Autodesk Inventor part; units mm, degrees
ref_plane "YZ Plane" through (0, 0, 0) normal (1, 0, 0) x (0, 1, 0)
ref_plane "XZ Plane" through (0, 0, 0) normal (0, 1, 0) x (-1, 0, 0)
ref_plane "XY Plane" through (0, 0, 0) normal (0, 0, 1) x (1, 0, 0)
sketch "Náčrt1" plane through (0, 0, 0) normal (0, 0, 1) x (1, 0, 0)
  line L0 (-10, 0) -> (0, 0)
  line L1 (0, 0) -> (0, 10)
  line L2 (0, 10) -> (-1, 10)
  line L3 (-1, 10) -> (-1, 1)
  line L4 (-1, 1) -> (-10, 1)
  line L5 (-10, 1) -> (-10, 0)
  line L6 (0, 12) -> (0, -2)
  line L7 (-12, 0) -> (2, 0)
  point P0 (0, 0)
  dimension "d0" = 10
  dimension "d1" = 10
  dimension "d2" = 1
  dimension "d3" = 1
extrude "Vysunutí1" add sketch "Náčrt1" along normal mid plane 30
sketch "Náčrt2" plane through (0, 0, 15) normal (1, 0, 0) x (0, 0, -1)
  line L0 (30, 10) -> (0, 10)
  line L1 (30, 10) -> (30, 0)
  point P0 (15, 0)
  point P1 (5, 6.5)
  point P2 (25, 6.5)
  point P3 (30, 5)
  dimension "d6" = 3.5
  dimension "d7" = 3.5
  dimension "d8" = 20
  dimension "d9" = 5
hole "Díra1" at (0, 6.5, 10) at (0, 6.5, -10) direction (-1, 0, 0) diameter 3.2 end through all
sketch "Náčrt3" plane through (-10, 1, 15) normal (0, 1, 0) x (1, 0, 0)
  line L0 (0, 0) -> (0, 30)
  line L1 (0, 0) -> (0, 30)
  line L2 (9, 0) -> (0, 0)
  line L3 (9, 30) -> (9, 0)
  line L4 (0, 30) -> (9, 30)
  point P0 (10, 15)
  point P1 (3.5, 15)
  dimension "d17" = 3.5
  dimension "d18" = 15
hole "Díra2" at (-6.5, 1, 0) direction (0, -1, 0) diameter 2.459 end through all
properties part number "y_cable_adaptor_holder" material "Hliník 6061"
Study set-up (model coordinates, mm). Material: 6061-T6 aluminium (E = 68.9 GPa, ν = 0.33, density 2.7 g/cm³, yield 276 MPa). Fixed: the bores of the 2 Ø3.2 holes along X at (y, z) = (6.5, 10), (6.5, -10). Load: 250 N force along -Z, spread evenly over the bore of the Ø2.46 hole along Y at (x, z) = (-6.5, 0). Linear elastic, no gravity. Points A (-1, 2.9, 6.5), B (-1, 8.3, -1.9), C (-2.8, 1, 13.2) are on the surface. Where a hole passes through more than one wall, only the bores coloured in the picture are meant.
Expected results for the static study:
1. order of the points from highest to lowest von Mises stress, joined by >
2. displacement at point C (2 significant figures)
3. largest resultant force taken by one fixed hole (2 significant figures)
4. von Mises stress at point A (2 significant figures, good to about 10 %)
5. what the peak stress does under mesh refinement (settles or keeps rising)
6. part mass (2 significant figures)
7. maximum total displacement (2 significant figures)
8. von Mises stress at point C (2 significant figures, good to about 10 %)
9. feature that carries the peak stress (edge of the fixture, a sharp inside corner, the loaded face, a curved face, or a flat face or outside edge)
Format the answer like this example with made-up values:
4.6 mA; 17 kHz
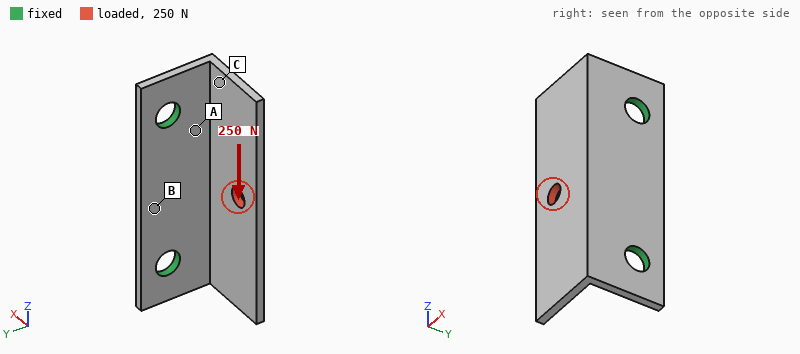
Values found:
A > C > B; 48 µm; 160 N; 68 MPa; keeps rising; 1.5 g; 99 µm; 40 MPa; edge of the fixture
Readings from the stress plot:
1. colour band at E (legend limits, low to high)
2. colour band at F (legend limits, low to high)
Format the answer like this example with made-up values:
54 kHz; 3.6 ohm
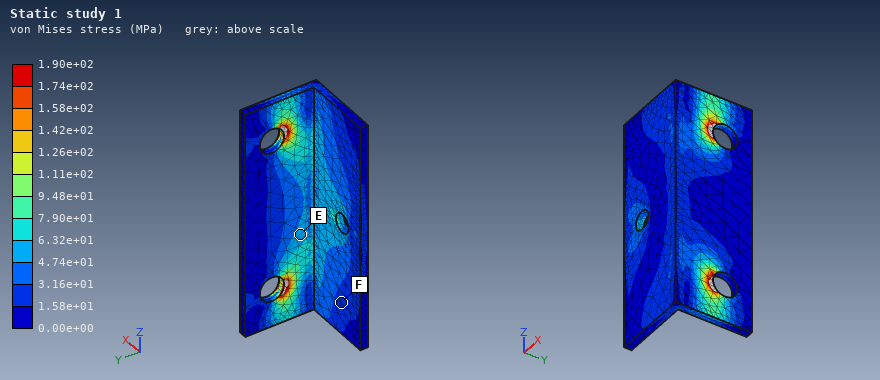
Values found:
4.74e+01 to 6.32e+01 MPa; 1.58e+01 to 3.16e+01 MPa
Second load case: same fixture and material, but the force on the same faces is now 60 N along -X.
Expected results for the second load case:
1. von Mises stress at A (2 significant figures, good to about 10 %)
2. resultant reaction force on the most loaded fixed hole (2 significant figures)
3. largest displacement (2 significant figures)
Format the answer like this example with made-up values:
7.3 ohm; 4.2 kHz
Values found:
27 MPa; 31 N; 55 µm
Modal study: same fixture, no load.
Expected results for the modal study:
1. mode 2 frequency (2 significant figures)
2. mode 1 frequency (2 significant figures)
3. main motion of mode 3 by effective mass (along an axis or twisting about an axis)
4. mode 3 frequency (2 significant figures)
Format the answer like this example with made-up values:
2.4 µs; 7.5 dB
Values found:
7200 Hz; 4800 Hz; along X; 13 kHz
